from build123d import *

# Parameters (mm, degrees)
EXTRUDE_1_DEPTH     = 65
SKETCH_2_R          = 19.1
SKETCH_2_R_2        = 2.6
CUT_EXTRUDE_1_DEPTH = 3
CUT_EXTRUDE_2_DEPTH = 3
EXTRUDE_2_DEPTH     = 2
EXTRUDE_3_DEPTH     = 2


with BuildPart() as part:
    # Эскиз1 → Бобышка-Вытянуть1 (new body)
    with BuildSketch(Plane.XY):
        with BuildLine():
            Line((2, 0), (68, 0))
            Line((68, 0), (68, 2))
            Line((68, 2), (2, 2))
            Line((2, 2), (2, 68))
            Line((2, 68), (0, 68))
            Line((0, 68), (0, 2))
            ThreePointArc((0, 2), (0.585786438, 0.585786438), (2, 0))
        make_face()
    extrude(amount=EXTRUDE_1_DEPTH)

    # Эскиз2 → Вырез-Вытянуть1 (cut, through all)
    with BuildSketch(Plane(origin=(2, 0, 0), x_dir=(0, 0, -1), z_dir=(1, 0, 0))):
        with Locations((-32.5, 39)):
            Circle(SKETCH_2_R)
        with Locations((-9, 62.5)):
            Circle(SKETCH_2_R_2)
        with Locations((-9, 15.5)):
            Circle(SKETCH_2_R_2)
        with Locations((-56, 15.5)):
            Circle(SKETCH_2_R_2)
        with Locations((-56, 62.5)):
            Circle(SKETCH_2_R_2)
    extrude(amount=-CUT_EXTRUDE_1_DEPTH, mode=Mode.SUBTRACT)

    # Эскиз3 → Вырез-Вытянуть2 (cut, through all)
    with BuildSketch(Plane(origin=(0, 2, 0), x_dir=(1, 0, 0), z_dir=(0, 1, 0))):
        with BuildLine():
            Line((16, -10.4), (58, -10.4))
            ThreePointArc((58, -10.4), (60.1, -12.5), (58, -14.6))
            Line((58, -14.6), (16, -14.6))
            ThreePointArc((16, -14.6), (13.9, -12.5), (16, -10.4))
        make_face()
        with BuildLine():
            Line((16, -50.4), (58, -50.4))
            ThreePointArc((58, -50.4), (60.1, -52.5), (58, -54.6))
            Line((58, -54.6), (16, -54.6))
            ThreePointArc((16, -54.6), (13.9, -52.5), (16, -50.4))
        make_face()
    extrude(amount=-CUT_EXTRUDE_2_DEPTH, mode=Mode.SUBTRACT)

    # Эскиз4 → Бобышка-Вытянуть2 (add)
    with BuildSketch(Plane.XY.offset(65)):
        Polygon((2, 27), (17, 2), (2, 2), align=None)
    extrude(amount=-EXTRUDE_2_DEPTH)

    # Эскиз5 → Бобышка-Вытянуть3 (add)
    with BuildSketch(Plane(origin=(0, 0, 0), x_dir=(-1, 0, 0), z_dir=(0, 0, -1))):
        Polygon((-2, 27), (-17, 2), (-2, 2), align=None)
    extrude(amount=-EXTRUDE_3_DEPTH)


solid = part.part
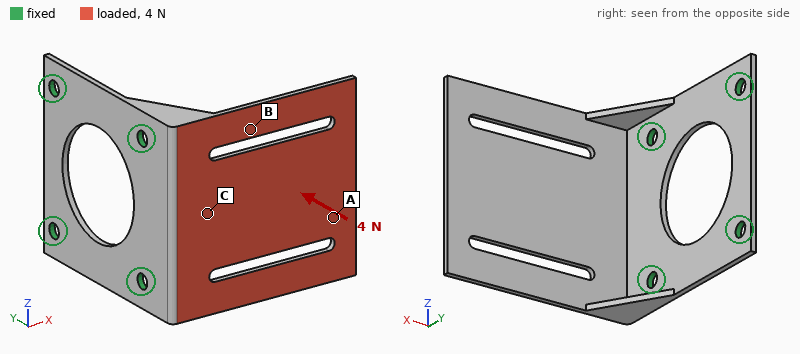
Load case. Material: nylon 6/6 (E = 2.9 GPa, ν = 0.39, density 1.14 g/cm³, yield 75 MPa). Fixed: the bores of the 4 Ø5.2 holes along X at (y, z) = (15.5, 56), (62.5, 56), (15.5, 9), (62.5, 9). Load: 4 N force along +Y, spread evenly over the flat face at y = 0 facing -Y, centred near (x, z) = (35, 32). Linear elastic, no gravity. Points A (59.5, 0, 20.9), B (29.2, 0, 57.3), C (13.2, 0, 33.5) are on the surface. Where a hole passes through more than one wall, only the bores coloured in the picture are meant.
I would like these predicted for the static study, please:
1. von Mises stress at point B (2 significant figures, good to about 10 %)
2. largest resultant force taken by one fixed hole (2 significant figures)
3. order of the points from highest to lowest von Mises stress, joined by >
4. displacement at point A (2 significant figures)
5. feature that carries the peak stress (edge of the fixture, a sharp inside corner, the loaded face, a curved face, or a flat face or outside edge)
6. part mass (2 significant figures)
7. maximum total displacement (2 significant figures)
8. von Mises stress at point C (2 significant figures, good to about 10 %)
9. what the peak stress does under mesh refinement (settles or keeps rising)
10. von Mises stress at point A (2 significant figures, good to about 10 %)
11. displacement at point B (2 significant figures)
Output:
1.9 MPa
2.5 N
B > C > A
0.99 mm
a sharp inside corner
17 g
1.2 mm
1.3 MPa
keeps rising
0.47 MPa
0.26 mm
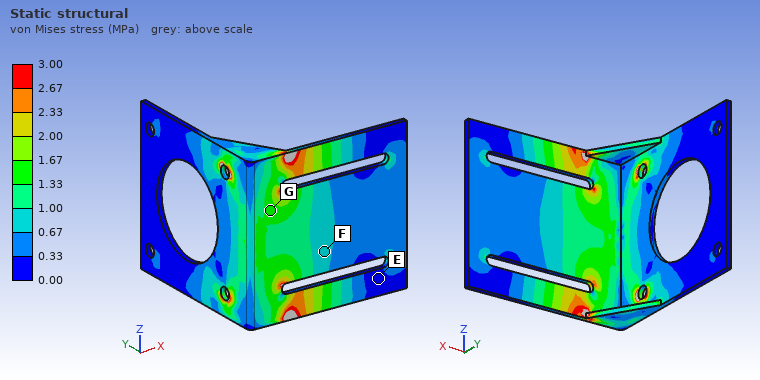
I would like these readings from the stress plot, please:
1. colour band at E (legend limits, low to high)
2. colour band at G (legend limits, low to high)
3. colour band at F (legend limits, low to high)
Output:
0.00 to 0.33 MPa
1.33 to 1.67 MPa
0.67 to 1.00 MPa
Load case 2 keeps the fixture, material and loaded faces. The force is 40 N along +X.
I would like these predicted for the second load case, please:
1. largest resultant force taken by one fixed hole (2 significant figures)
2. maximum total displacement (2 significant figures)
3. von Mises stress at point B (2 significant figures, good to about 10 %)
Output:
22 N
1.3 mm
1.1 MPa
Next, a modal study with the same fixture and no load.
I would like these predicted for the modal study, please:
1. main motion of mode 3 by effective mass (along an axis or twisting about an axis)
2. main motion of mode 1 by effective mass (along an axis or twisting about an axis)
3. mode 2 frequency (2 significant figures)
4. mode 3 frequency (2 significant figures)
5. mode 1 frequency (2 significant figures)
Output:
along Z
along Y
310 Hz
520 Hz
120 Hz
